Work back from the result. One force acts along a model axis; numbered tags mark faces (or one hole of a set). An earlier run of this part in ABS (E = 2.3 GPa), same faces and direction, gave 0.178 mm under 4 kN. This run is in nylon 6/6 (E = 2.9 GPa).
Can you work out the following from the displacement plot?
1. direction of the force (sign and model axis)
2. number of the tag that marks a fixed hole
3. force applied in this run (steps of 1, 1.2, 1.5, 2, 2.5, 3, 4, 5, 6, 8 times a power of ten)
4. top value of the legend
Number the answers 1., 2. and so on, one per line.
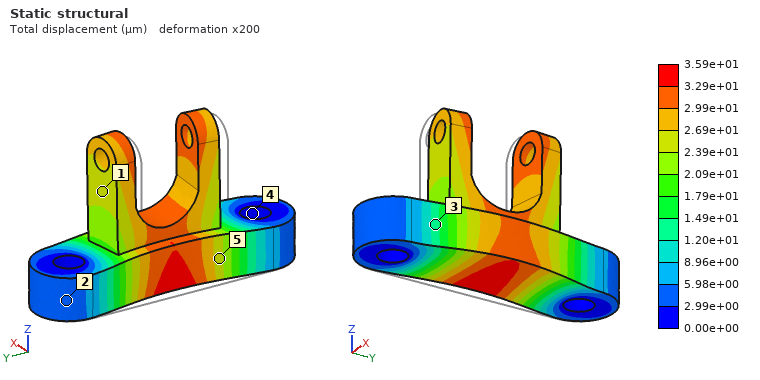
1. +X
2. 4
3. 1 kN
4. 3.59e+01 µm
